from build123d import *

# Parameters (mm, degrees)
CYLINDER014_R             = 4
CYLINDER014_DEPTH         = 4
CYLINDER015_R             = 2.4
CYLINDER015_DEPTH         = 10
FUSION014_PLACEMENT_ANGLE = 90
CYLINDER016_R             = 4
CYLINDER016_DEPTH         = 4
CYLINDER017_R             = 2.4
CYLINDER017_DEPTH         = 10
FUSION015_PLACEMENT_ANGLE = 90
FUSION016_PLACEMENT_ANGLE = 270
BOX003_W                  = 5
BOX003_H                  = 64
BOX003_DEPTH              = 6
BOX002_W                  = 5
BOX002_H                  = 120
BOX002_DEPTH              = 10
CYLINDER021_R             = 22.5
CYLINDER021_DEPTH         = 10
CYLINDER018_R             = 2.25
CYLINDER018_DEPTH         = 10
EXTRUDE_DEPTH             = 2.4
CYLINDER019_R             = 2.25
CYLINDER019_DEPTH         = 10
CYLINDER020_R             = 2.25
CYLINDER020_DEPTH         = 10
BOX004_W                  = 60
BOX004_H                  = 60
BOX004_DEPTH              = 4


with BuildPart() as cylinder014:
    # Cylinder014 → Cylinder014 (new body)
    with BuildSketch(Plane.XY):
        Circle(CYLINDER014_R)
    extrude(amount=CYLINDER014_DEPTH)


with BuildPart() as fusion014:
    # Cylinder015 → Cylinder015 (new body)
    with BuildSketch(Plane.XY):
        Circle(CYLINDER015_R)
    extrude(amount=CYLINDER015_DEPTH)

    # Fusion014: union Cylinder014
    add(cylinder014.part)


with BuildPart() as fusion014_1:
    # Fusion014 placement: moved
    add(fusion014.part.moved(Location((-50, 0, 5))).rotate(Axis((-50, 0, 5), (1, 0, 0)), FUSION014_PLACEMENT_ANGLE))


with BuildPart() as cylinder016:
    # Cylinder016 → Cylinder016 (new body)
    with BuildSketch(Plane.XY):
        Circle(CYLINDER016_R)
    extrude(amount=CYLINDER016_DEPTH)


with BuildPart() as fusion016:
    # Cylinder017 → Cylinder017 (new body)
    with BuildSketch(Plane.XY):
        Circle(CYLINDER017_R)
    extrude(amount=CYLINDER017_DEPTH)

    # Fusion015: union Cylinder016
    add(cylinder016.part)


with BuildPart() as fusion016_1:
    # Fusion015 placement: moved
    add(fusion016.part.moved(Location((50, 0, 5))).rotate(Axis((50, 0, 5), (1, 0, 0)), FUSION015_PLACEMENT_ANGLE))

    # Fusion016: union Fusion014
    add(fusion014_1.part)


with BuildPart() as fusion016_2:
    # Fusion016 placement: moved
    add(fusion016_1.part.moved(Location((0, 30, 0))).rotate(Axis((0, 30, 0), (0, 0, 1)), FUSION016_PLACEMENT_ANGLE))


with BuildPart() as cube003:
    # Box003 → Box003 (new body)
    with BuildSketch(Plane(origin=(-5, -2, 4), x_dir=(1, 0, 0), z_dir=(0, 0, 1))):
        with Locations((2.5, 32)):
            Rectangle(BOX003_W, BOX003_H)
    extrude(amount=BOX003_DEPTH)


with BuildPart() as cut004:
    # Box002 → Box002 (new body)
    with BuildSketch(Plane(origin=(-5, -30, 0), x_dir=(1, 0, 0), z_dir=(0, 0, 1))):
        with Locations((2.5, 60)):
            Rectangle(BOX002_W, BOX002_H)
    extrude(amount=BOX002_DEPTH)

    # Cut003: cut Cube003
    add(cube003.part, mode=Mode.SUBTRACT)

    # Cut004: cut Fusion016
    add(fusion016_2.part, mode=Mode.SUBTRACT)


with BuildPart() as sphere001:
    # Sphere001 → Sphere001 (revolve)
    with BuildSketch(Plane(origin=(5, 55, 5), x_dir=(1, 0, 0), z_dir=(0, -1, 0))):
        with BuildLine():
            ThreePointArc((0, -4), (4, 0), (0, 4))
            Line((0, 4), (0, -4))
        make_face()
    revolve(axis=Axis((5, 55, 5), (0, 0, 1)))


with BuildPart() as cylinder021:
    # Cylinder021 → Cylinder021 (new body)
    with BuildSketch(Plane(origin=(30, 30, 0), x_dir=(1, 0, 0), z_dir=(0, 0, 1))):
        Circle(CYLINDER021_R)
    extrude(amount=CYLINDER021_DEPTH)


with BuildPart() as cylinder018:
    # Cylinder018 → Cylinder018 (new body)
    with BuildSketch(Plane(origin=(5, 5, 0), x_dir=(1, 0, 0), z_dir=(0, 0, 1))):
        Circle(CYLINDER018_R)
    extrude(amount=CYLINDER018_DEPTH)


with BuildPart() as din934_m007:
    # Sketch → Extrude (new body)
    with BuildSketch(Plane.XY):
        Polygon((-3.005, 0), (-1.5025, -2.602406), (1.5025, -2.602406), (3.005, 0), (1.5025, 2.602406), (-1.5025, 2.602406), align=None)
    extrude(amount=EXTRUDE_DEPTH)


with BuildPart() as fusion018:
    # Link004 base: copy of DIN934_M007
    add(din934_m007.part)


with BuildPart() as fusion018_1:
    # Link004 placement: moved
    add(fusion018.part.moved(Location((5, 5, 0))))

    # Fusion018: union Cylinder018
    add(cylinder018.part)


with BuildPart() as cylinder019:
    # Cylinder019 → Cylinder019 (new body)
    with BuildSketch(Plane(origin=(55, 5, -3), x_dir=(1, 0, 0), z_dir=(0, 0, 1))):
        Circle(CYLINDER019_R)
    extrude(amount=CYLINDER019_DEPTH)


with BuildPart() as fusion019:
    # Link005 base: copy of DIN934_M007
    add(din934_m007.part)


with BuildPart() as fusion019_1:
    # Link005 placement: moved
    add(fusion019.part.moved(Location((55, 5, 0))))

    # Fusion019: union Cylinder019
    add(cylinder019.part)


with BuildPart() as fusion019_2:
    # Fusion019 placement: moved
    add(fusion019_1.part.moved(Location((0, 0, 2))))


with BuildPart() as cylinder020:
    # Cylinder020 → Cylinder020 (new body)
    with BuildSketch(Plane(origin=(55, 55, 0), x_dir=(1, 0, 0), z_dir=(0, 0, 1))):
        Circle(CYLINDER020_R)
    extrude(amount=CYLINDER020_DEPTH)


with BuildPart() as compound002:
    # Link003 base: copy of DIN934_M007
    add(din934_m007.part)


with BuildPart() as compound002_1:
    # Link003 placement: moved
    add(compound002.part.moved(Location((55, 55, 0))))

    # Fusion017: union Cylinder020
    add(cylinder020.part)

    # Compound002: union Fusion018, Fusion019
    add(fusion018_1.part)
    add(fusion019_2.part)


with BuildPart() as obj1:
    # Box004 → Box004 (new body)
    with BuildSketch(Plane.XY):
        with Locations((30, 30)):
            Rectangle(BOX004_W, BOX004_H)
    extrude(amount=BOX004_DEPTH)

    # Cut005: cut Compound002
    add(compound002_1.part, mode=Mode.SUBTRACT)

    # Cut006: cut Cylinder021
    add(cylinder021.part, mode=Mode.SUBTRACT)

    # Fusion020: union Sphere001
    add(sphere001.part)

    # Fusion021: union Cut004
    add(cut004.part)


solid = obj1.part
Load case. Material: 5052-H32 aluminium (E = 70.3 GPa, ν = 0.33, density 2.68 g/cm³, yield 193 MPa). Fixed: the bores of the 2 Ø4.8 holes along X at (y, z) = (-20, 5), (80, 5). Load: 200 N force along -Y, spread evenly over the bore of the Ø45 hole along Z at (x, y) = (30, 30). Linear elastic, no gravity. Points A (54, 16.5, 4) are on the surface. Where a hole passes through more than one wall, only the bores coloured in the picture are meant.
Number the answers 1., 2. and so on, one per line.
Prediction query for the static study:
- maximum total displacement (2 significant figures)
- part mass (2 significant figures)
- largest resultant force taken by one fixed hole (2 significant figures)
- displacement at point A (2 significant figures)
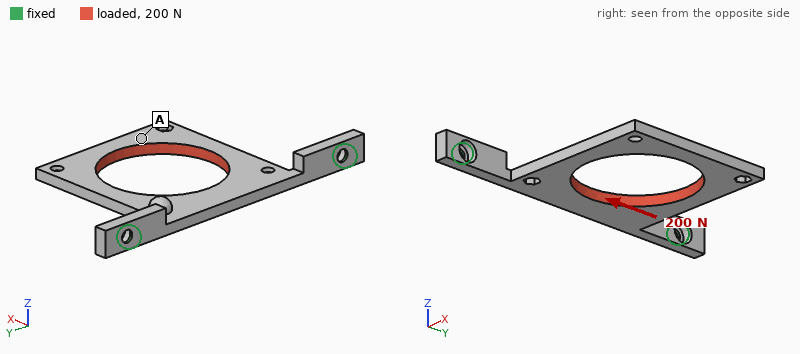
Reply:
1. 75 µm
2. 31 g
3. 130 N
4. 64 µm
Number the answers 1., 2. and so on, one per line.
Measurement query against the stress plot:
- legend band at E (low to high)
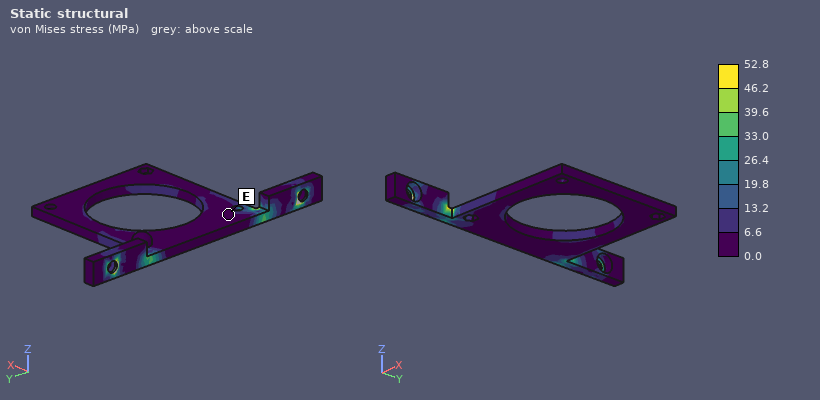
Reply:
1. 0.0 to 6.6 MPa
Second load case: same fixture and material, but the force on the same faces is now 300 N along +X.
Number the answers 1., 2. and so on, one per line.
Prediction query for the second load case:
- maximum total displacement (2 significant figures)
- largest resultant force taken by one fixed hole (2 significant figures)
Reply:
1. 0.15 mm
2. 310 N
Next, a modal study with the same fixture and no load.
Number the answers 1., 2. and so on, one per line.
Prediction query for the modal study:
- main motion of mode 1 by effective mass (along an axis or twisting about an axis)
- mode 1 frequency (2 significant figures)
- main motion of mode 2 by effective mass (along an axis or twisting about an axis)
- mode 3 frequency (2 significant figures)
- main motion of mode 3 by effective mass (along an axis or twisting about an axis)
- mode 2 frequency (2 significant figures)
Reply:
1. along Z
2. 370 Hz
3. twisting about X
4. 1900 Hz
5. along Y
6. 1400 Hz
